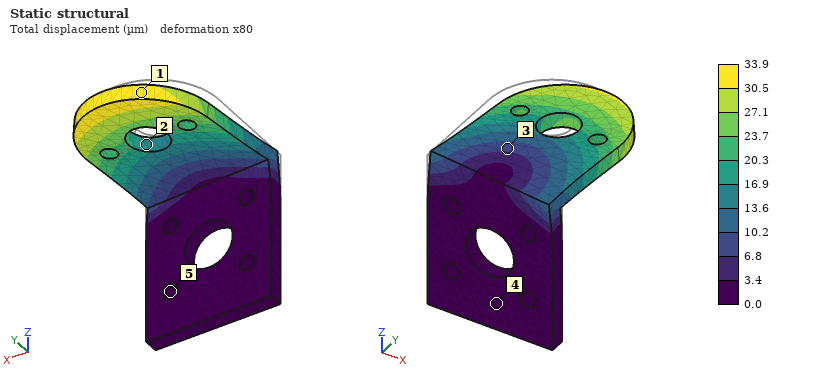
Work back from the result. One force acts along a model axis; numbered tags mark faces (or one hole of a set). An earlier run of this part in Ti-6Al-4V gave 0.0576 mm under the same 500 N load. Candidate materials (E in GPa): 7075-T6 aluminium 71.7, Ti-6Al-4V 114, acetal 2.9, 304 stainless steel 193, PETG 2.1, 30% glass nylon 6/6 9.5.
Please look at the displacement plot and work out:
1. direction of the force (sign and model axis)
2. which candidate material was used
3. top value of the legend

+X
304 stainless steel
33.9 µm
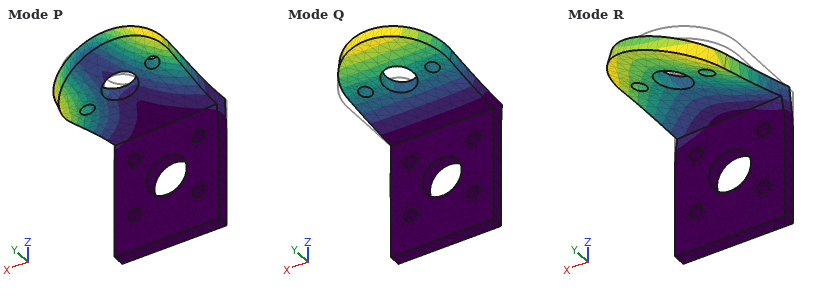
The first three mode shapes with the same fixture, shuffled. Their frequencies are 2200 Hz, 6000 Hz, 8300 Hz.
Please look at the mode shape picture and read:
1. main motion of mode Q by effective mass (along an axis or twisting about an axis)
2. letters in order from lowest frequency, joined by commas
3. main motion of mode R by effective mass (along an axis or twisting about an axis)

along Z
Q, R, P
along X
